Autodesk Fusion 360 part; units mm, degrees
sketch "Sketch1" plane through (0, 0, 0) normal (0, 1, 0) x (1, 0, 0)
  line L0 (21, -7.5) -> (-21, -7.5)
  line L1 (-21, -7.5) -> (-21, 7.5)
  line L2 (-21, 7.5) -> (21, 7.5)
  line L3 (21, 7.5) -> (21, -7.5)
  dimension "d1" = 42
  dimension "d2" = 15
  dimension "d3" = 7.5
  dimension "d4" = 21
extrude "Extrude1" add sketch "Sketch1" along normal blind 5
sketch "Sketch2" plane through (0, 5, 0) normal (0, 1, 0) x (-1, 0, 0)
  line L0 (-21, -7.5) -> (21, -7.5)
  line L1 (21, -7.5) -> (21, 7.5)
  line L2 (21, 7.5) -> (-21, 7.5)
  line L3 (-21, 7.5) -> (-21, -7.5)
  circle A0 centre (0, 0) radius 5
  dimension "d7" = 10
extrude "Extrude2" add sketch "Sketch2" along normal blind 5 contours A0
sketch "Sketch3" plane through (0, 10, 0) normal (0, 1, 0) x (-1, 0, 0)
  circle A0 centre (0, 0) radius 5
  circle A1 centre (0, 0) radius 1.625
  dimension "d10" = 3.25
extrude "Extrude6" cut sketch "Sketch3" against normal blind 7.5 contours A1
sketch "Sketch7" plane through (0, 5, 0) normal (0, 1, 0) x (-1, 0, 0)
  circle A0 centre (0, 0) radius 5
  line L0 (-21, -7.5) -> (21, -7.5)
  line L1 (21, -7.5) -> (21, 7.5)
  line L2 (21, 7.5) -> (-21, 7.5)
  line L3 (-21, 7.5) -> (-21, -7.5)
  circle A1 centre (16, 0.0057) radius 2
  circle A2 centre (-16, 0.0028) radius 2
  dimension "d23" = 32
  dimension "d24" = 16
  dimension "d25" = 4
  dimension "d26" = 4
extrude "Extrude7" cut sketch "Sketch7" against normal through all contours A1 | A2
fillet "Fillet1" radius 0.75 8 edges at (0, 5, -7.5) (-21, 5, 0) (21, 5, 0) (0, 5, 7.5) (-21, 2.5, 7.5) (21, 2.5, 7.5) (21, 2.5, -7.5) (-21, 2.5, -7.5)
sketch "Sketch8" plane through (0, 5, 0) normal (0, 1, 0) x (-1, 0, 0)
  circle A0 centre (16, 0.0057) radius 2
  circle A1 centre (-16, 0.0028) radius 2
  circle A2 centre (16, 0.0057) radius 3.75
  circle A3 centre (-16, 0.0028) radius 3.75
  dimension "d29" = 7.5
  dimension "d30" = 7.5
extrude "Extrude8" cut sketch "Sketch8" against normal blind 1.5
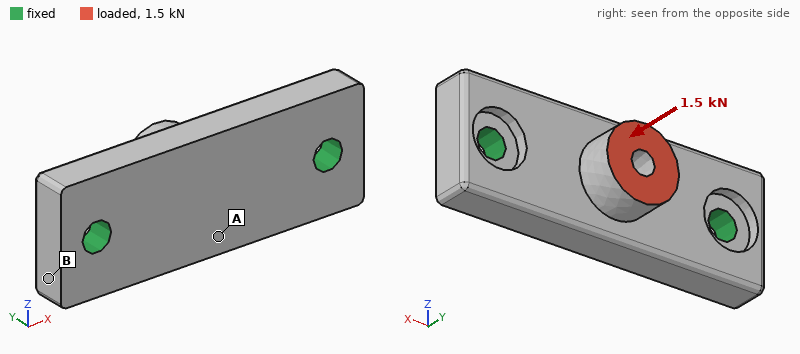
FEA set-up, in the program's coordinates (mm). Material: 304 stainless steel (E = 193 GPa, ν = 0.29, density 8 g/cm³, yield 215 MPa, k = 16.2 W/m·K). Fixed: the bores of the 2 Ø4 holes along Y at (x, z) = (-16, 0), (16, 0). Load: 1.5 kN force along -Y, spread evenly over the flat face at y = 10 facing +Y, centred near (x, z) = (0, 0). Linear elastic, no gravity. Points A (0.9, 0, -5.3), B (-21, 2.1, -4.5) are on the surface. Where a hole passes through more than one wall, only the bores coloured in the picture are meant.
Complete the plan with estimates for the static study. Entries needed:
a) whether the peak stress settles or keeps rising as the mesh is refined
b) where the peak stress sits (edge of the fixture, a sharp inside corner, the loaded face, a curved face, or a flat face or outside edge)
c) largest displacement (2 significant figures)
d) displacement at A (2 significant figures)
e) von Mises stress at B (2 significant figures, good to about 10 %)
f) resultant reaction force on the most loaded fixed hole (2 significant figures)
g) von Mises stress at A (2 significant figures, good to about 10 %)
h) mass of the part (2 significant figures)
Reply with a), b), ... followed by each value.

a) keeps rising
b) edge of the fixture
c) 10 µm
d) 9.9 µm
e) 15 MPa
f) 890 N
g) 51 MPa
h) 26 g
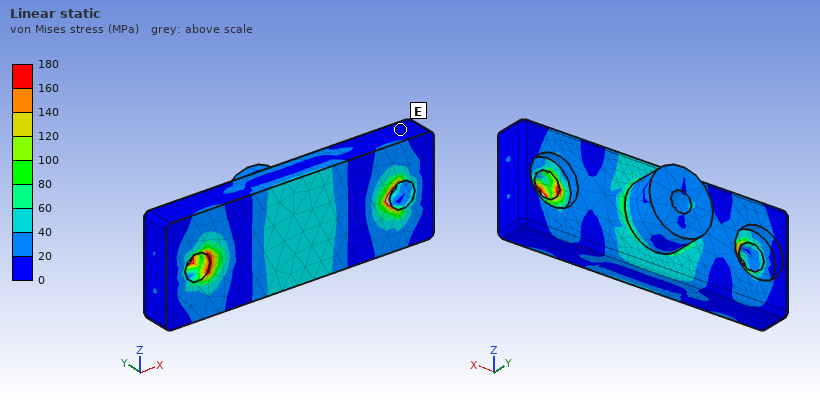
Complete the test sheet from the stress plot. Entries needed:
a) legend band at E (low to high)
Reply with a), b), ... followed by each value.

a) 0 to 20 MPa
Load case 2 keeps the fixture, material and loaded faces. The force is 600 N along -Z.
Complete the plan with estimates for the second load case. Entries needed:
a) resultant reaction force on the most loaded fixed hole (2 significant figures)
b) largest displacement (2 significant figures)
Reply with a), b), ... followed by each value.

a) 300 N
b) 12 µm
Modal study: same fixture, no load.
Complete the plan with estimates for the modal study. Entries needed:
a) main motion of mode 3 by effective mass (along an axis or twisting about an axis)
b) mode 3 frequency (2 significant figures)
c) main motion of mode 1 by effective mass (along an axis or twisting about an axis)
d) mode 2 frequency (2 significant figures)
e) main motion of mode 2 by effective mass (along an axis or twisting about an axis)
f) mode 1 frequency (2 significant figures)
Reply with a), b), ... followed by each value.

a) along Z
b) 29 kHz
c) along Y
d) 19 kHz
e) along Z
f) 18 kHz
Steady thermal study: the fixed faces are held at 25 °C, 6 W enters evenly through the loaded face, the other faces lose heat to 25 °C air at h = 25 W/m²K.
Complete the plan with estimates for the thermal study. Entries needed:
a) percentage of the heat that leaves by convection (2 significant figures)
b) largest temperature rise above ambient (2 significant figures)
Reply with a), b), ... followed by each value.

a) 15 %
b) 63 K
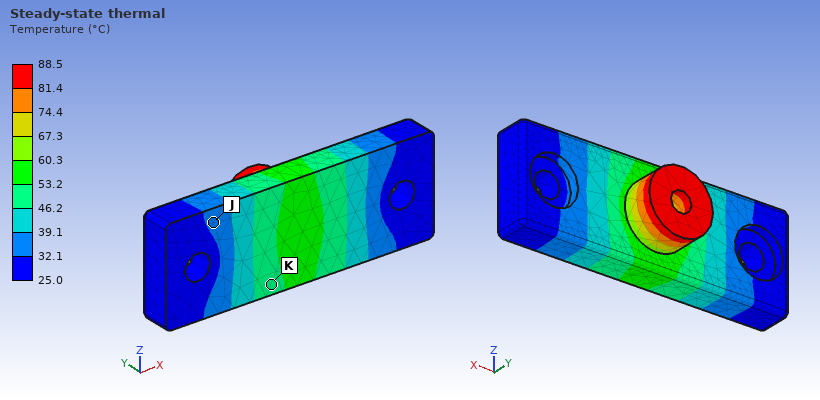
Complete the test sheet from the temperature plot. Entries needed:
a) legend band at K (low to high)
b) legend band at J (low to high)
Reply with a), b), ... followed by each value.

a) 46.2 to 53.2 °C
b) 32.1 to 39.1 °C
